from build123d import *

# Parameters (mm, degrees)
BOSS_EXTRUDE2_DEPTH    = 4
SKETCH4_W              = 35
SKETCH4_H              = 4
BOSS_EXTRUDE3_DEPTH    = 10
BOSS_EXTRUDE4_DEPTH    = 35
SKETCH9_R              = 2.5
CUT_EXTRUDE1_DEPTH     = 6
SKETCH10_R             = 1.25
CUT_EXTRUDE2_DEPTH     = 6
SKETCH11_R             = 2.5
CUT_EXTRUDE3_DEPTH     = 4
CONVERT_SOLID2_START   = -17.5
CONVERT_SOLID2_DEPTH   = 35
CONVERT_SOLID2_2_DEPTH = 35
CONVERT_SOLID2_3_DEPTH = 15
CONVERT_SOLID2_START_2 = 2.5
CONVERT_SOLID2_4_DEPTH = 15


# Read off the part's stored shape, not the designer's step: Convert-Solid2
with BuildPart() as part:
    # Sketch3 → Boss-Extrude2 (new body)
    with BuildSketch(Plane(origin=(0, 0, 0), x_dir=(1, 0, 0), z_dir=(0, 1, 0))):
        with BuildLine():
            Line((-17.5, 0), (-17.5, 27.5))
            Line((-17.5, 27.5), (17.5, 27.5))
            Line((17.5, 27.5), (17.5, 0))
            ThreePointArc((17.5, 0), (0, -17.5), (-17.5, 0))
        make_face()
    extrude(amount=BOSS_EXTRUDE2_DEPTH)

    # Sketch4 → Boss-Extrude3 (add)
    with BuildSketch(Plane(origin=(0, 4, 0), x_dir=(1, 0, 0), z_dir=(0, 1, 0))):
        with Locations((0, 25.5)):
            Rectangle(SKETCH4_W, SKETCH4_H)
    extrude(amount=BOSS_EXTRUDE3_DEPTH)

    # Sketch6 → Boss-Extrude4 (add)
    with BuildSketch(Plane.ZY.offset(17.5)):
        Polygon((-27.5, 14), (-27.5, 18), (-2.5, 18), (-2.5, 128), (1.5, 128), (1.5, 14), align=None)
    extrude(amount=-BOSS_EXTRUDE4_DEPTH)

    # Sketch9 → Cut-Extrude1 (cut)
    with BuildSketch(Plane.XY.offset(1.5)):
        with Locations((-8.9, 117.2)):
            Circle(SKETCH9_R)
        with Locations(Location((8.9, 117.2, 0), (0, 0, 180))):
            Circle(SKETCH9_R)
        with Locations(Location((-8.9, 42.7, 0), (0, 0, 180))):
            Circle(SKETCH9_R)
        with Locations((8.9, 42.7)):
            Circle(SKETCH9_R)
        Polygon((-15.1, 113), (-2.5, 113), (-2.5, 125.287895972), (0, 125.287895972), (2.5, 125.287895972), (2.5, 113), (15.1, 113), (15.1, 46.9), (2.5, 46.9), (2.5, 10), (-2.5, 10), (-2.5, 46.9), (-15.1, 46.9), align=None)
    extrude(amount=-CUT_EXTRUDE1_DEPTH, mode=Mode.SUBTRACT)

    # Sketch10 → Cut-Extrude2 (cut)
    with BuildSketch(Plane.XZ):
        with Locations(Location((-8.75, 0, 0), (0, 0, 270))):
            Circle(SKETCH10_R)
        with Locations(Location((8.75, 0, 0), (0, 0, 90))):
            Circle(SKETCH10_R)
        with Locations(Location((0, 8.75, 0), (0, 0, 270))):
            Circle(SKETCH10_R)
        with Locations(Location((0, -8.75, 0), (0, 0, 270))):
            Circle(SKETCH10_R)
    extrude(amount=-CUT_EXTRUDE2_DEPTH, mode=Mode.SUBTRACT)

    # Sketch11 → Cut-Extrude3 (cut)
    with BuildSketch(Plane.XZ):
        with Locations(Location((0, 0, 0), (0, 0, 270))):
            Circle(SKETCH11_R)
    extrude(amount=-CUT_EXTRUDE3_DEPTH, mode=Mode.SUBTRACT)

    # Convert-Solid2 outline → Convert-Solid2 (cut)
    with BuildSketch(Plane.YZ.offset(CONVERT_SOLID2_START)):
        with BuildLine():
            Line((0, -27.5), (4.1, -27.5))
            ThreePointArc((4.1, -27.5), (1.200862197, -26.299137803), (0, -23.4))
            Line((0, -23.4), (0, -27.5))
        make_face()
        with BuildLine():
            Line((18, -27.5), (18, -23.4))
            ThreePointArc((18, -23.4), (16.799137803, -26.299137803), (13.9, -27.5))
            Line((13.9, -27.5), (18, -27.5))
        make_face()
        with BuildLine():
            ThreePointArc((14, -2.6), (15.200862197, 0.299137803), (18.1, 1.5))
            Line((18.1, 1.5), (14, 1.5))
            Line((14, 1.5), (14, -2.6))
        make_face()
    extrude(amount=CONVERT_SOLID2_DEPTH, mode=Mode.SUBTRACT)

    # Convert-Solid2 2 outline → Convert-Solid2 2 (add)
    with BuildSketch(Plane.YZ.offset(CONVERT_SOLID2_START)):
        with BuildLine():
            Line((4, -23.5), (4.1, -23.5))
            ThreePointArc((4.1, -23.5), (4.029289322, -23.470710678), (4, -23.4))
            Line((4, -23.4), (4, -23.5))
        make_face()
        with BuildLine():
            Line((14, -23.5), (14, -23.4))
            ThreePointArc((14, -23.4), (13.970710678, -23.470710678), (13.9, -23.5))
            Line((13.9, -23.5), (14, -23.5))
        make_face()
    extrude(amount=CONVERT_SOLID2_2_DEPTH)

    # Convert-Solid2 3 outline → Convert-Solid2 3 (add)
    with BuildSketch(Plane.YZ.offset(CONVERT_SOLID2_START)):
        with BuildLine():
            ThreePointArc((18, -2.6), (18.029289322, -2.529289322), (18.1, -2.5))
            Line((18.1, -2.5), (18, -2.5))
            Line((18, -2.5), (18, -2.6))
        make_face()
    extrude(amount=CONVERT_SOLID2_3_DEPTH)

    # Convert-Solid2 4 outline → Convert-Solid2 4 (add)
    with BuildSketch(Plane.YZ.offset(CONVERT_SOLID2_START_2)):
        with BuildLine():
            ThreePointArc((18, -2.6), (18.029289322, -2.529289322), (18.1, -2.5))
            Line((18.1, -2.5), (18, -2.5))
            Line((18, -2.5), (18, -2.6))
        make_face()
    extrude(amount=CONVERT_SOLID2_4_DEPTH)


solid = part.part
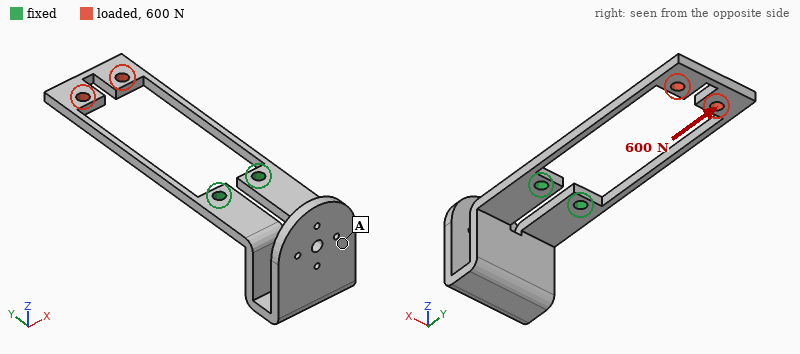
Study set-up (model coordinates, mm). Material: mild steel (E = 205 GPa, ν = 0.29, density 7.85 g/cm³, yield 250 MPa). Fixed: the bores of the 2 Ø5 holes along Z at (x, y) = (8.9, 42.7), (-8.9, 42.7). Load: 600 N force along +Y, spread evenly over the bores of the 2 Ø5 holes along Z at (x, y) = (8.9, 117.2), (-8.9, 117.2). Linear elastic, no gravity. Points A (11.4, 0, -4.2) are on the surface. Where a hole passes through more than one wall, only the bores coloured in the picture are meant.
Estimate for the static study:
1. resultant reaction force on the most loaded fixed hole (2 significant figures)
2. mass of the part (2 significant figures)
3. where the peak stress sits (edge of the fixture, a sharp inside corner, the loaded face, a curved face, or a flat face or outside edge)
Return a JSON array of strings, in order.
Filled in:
["300 N", "130 g", "a flat face or outside edge"]
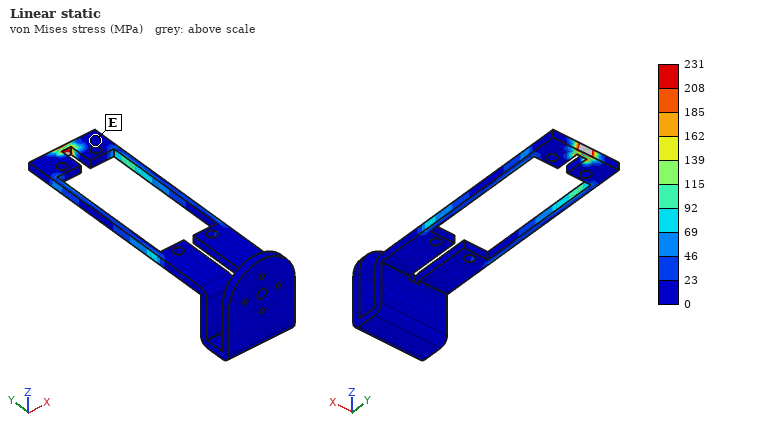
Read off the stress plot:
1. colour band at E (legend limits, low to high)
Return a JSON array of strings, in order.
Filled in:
["0 to 23 MPa"]
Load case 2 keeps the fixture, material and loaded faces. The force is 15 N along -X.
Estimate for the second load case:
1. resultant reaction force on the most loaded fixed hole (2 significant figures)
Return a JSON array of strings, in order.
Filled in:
["21 N"]
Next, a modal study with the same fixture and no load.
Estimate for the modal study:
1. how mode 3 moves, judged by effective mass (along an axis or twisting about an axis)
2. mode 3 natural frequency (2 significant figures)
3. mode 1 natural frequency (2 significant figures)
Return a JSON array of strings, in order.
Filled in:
["along Z", "650 Hz", "240 Hz"]
